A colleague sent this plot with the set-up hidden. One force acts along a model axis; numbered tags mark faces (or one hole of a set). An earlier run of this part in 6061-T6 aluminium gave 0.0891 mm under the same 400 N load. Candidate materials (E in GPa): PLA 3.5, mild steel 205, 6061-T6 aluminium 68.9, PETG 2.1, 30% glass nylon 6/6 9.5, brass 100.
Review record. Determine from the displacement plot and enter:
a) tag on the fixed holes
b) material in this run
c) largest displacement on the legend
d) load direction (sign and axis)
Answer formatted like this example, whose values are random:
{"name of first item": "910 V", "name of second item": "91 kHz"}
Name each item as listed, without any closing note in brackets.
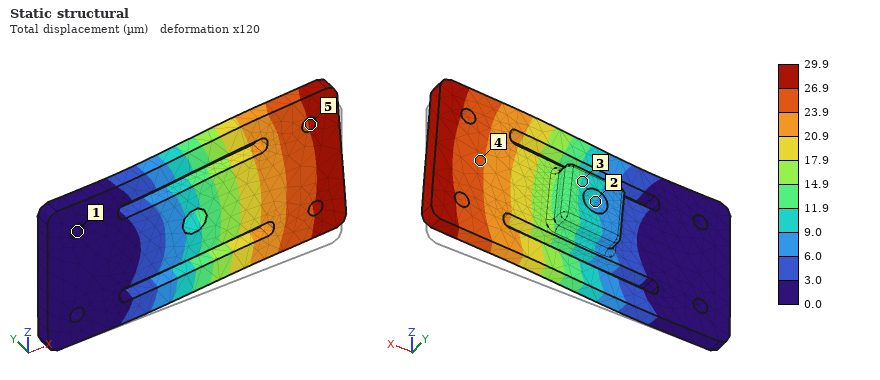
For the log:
{"tag on the fixed holes": "1", "material in this run": "mild steel", "largest displacement on the legend": "29.9 µm", "load direction": "+Z"}
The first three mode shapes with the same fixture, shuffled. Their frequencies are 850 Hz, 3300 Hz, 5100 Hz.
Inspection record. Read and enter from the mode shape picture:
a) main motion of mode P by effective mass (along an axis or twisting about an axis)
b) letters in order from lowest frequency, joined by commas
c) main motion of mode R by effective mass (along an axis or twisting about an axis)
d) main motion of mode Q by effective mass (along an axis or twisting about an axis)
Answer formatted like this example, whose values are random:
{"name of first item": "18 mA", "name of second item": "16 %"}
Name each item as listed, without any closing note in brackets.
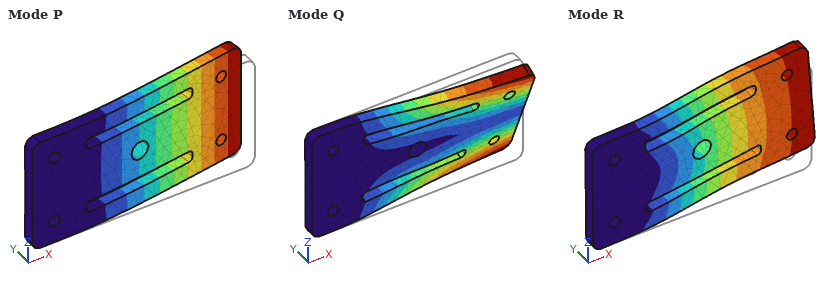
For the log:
{"main motion of mode P by effective mass": "along Y", "letters in order from lowest frequency, joined by commas": "P, Q, R", "main motion of mode R by effective mass": "along Z", "main motion of mode Q by effective mass": "twisting about X"}
